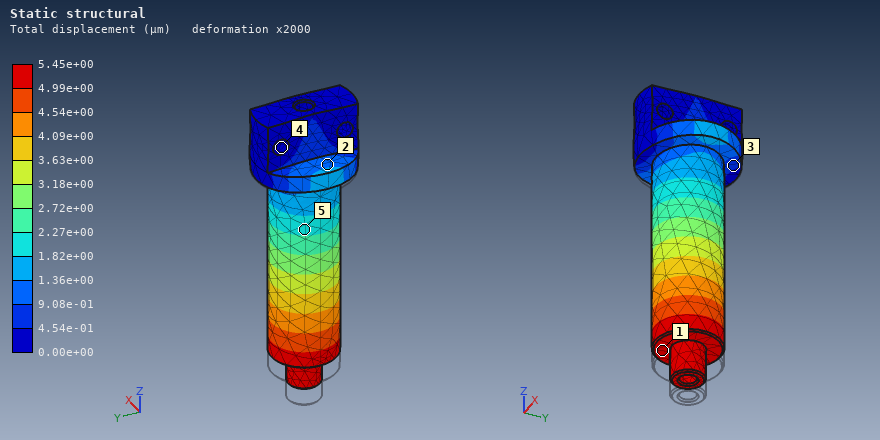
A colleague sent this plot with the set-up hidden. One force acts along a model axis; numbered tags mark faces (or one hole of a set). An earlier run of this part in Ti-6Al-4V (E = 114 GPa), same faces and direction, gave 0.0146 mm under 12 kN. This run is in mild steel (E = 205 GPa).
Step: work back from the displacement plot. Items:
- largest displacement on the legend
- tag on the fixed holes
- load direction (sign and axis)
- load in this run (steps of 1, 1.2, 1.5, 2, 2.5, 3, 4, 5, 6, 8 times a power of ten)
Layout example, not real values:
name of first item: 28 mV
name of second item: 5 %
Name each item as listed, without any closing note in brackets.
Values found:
largest displacement on the legend: 5.45e+00 µm
tag on the fixed holes: 4
load direction: +Z
load in this run: 8 kN
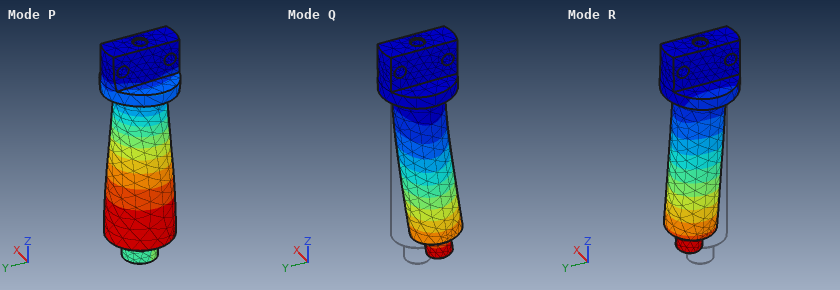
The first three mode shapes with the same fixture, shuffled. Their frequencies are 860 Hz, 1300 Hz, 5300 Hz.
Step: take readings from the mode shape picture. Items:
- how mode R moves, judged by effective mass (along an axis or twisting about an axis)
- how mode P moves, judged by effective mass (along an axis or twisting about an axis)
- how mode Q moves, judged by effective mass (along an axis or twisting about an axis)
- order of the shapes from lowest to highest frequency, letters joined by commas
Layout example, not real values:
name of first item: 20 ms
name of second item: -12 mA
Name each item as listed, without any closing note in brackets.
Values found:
how mode R moves, judged by effective mass: along X
how mode P moves, judged by effective mass: twisting about Z
how mode Q moves, judged by effective mass: along Y
order of the shapes from lowest to highest frequency, letters joined by commas: R, Q, P
